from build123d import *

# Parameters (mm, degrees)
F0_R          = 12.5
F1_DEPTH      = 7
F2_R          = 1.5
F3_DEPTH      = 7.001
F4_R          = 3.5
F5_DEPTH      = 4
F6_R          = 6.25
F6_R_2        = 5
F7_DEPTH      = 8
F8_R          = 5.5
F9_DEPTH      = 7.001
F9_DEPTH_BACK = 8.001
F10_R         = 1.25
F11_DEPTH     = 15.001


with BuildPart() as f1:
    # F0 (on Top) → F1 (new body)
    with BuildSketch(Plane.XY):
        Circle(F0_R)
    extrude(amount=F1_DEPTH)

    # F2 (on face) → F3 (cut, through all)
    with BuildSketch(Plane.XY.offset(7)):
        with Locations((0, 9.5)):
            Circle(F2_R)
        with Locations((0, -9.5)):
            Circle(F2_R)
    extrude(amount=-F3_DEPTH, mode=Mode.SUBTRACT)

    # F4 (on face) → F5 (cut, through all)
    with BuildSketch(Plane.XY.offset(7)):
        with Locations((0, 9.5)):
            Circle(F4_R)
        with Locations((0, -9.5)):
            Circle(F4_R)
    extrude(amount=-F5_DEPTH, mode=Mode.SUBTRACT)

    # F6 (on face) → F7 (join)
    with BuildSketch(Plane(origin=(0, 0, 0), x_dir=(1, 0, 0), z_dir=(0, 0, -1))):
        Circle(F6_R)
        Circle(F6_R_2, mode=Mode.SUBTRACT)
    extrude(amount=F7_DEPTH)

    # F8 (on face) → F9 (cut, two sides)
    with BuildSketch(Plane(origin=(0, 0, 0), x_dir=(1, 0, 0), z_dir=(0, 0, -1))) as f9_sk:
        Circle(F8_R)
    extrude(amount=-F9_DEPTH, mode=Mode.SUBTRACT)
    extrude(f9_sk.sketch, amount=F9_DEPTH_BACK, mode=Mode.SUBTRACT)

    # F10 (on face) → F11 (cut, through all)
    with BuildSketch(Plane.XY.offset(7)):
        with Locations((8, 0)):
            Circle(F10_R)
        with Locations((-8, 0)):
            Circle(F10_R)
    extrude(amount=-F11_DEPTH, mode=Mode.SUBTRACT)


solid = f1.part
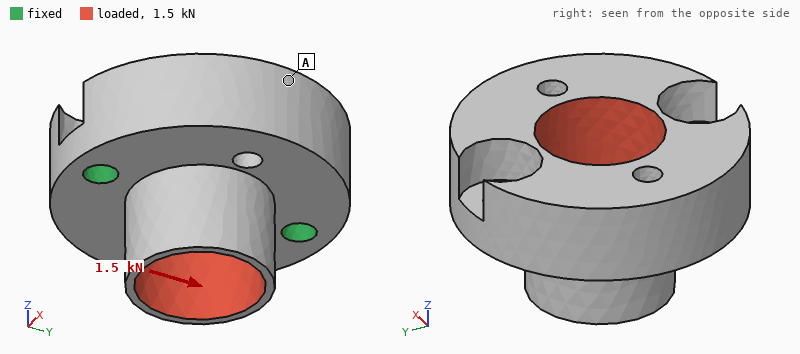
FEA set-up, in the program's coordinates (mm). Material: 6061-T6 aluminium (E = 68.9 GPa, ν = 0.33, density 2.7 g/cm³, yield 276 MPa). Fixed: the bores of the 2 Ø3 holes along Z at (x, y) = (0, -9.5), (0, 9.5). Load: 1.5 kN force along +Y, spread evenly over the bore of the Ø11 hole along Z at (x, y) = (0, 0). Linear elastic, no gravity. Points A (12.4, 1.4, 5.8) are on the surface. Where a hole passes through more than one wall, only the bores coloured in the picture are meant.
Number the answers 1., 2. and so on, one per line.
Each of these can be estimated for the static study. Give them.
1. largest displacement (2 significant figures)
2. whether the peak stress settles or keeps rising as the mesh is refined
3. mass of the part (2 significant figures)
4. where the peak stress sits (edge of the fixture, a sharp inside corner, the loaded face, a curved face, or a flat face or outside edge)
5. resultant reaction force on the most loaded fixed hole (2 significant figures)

1. 18 µm
2. keeps rising
3. 7.0 g
4. edge of the fixture
5. 780 N
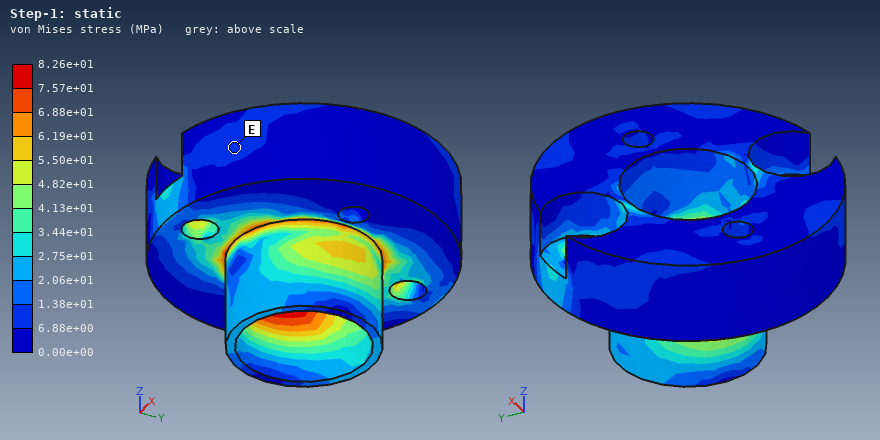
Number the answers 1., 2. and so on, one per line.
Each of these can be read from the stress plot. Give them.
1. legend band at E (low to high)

1. 6.88e+00 to 1.38e+01 MPa
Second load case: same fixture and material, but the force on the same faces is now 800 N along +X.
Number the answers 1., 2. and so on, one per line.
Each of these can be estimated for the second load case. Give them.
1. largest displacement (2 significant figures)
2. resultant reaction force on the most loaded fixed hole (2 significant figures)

1. 16 µm
2. 400 N
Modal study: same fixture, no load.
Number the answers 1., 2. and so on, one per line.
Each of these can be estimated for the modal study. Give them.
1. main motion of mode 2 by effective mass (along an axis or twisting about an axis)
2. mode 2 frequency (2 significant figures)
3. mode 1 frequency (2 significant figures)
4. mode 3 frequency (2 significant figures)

1. along Z
2. 20 kHz
3. 12 kHz
4. 32 kHz
